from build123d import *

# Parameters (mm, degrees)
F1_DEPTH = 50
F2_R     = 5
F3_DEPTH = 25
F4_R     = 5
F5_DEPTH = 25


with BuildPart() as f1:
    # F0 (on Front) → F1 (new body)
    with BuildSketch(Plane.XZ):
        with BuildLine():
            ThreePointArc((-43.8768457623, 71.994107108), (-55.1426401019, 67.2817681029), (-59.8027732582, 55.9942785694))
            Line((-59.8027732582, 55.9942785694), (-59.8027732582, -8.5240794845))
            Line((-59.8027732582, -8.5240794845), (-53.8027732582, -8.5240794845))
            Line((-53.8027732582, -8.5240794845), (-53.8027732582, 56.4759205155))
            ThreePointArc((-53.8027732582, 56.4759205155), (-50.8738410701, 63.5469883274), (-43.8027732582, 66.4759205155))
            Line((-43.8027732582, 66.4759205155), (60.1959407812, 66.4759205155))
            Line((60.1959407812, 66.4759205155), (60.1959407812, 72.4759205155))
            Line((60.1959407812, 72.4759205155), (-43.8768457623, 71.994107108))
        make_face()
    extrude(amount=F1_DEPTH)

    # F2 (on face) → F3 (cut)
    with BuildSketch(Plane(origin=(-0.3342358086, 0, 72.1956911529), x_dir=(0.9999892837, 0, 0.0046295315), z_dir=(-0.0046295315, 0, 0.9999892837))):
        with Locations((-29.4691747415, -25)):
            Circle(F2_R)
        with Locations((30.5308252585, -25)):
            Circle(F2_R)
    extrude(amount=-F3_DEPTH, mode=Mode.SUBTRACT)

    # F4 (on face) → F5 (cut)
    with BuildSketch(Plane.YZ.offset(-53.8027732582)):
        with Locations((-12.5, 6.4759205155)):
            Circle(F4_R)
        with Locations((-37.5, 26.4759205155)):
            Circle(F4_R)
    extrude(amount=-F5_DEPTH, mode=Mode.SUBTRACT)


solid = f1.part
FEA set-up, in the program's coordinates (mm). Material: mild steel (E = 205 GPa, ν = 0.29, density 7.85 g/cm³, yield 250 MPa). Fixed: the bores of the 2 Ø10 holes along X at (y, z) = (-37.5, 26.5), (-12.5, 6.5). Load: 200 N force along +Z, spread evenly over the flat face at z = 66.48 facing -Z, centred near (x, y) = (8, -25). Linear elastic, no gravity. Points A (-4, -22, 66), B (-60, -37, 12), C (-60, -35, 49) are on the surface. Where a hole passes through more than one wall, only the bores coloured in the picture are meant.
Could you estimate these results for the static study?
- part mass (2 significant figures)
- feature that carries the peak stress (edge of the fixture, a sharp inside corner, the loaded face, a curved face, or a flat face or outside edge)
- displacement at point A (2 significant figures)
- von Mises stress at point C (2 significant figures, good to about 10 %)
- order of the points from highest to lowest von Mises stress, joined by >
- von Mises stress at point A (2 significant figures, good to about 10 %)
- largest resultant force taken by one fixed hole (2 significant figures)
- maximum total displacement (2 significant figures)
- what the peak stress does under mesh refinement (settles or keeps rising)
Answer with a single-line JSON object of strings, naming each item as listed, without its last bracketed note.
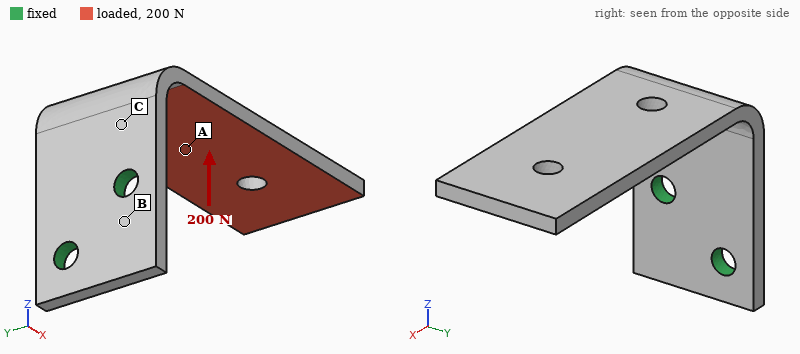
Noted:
{"part mass": "420 g", "feature that carries the peak stress": "edge of the fixture", "displacement at point A": "0.23 mm", "von Mises stress at point C": "39 MPa", "order of the points from highest to lowest von Mises stress, joined by >": "C > A > B", "von Mises stress at point A": "14 MPa", "largest resultant force taken by one fixed hole": "210 N", "maximum total displacement": "0.61 mm", "what the peak stress does under mesh refinement": "keeps rising"}
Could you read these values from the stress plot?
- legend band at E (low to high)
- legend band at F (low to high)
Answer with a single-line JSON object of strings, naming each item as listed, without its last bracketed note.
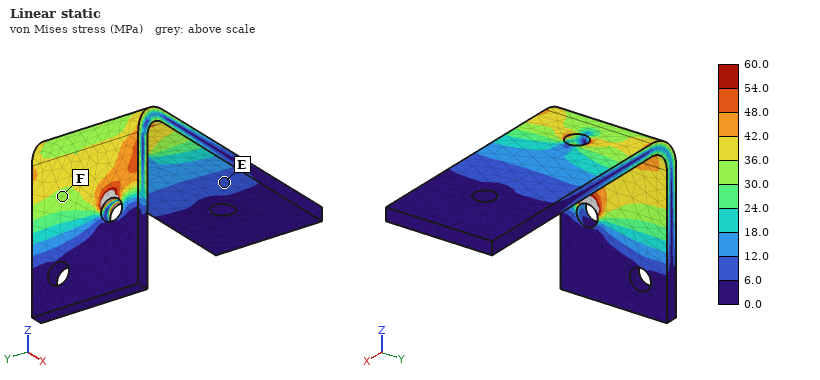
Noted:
{"legend band at E": "6.0 to 12.0 MPa", "legend band at F": "30.0 to 36.0 MPa"}
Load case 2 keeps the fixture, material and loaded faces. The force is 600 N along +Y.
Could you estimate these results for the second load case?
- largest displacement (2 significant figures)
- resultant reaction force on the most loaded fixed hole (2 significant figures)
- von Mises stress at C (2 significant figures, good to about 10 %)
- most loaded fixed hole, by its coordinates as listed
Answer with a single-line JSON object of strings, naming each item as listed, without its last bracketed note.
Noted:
{"largest displacement": "0.64 mm", "resultant reaction force on the most loaded fixed hole": "1.0 kN", "von Mises stress at C": "110 MPa", "most loaded fixed hole, by its coordinates as listed": "(-37.5, 26.5)"}
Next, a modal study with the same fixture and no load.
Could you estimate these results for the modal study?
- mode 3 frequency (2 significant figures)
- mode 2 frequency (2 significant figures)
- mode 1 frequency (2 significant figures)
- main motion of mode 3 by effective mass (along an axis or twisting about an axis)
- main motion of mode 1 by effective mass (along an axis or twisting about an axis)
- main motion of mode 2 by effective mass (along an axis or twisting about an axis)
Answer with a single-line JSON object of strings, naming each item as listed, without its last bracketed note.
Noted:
{"mode 3 frequency": "1000 Hz", "mode 2 frequency": "400 Hz", "mode 1 frequency": "230 Hz", "main motion of mode 3 by effective mass": "along X", "main motion of mode 1 by effective mass": "along Z", "main motion of mode 2 by effective mass": "along Y"}
